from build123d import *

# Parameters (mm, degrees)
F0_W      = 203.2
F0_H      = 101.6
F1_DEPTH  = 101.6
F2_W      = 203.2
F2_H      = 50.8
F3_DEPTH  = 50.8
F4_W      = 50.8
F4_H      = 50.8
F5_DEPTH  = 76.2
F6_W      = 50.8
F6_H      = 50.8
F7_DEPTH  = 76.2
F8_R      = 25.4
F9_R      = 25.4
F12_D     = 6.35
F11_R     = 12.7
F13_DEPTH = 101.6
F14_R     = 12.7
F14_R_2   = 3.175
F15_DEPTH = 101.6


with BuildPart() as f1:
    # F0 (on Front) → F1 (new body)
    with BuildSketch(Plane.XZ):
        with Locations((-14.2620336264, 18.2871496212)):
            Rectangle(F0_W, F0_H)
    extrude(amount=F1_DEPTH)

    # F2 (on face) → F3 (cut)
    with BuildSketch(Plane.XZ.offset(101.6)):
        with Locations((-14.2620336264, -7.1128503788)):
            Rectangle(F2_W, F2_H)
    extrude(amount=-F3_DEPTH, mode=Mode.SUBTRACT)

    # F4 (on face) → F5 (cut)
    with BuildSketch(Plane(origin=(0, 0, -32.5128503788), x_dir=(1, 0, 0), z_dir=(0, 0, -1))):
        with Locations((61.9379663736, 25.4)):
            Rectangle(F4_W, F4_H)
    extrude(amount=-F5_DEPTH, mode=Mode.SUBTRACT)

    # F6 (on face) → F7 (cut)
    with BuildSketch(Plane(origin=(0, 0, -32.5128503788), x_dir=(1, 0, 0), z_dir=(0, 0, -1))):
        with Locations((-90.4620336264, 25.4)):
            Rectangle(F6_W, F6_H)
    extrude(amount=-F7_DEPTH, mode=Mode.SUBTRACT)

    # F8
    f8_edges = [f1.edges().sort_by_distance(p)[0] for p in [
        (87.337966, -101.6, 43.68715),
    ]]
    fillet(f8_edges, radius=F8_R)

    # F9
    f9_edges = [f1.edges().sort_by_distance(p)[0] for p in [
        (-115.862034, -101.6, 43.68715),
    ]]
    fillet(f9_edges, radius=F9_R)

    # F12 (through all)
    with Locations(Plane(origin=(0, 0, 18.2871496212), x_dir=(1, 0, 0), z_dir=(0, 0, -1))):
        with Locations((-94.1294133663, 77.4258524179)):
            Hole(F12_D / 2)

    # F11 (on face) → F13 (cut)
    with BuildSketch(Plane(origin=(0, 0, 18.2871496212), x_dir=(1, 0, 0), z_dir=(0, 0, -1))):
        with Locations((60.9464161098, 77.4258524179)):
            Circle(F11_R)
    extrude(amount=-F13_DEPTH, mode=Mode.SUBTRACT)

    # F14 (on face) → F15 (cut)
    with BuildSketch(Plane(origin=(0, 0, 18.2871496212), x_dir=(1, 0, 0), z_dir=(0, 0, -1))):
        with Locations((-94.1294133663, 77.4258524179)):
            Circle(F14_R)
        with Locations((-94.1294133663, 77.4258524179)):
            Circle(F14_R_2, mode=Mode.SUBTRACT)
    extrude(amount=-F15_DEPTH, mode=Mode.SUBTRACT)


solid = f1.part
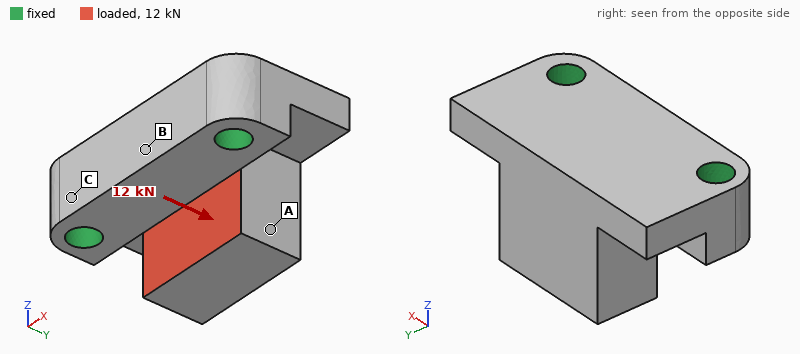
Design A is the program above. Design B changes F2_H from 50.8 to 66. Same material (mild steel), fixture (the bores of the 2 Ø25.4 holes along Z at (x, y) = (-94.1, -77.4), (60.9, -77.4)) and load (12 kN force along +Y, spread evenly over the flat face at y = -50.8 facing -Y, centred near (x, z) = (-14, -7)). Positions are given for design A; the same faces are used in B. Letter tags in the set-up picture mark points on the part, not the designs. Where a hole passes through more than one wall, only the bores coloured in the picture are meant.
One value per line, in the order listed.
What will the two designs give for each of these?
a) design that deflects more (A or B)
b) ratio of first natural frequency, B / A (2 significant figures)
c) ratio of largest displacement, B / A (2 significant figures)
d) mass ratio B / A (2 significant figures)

B
0.85
1.4
0.94
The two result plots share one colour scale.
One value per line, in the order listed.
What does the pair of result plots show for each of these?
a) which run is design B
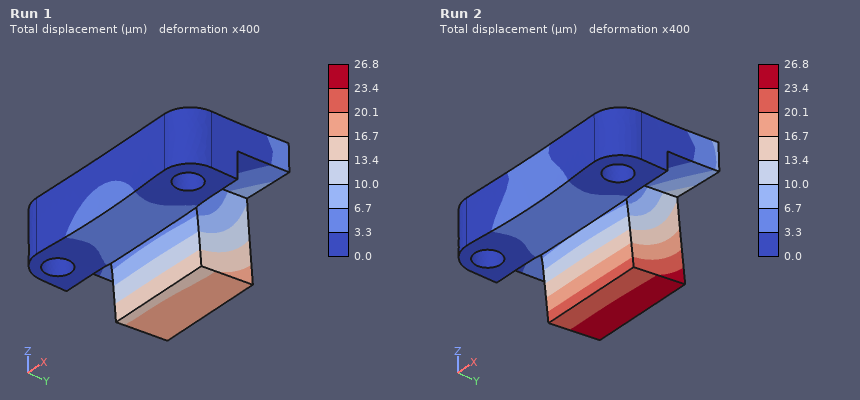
Run 2
